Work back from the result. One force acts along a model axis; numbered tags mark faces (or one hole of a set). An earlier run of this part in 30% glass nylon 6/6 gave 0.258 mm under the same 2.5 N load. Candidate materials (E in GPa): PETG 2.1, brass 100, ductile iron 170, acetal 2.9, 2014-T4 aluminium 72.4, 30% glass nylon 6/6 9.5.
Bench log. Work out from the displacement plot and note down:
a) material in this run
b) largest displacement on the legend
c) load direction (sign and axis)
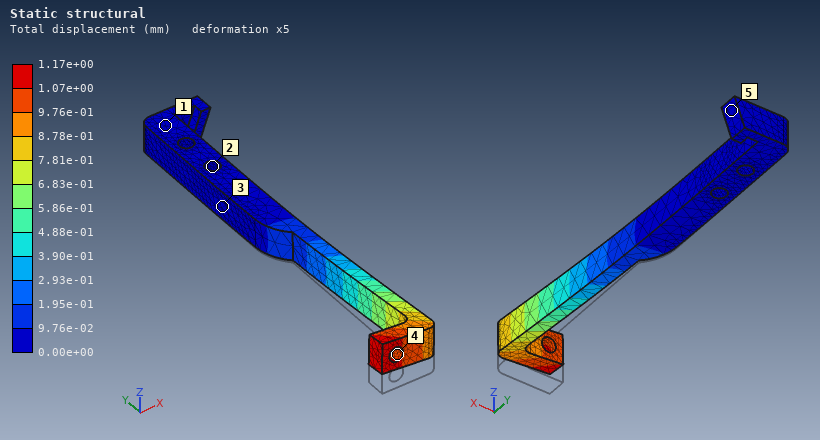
PETG
1.17e+00 mm
+Z
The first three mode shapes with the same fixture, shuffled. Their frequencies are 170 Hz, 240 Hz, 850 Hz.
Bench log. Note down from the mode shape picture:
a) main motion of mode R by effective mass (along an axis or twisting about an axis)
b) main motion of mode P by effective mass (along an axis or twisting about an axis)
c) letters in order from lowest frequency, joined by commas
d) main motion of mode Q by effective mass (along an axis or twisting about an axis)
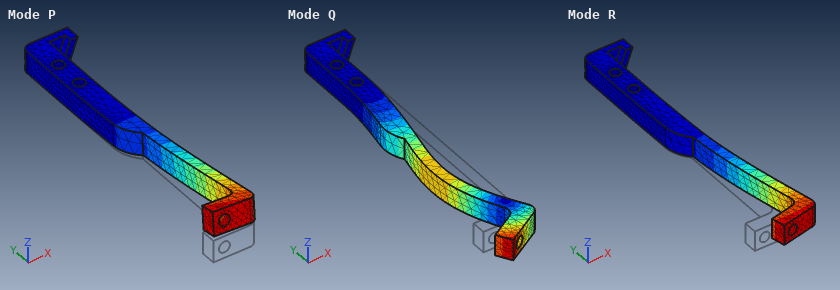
along X
along Z
R, P, Q
along X
